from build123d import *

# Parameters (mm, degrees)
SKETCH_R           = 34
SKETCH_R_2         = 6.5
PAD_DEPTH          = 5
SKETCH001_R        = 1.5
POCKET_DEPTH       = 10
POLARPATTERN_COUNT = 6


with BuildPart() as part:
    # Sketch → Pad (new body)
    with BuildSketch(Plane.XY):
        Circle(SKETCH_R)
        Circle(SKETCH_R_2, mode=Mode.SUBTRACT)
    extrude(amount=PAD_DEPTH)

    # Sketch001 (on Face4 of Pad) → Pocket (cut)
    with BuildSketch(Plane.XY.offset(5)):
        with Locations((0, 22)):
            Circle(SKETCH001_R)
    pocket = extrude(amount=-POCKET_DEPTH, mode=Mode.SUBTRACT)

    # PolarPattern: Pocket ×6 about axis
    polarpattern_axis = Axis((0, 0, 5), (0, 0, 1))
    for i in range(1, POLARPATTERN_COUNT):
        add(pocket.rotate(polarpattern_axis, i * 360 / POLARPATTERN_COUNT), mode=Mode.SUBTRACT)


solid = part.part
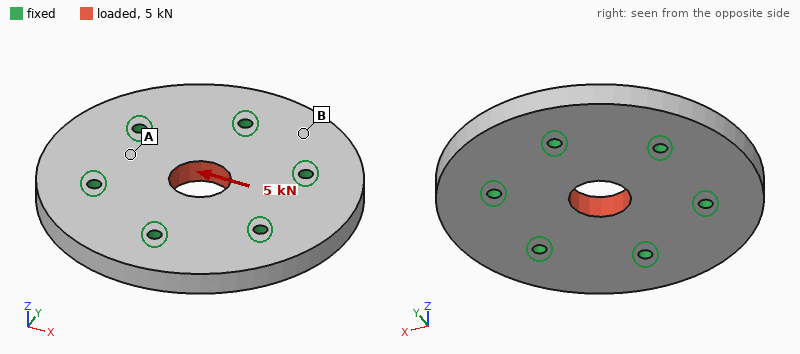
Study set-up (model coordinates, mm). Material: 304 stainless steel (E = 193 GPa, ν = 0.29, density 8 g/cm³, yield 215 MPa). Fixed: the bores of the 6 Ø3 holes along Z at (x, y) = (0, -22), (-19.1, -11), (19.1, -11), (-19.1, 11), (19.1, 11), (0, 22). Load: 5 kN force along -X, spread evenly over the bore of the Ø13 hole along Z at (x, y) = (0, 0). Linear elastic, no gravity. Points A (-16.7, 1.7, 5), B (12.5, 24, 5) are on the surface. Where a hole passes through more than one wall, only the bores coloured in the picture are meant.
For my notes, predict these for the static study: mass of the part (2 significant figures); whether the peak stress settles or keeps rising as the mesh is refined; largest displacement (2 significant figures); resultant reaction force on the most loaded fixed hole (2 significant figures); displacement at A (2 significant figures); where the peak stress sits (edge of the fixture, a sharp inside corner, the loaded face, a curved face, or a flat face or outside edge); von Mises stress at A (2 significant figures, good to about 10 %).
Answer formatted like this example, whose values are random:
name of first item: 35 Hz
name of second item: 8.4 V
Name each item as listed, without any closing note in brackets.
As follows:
mass of the part: 140 g
whether the peak stress settles or keeps rising as the mesh is refined: keeps rising
largest displacement: 1.9 µm
resultant reaction force on the most loaded fixed hole: 1.1 kN
displacement at A: 0.92 µm
where the peak stress sits: edge of the fixture
von Mises stress at A: 11 MPa
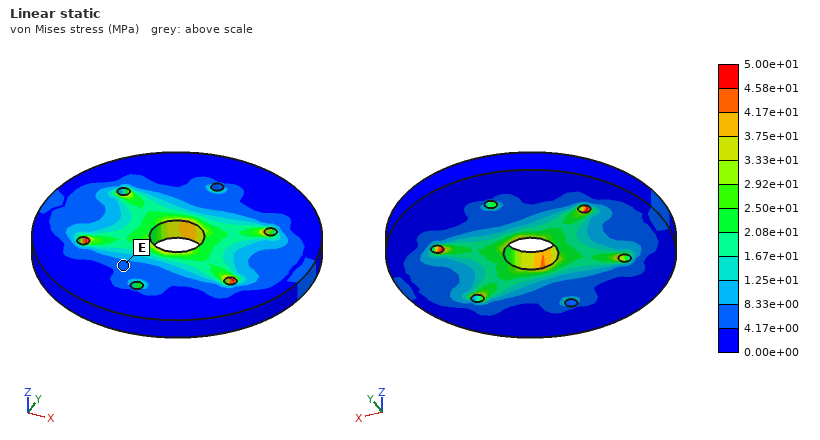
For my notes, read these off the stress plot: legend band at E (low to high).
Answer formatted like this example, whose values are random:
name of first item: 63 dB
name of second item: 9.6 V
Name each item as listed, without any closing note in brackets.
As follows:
legend band at E: 4.17e+00 to 8.33e+00 MPa
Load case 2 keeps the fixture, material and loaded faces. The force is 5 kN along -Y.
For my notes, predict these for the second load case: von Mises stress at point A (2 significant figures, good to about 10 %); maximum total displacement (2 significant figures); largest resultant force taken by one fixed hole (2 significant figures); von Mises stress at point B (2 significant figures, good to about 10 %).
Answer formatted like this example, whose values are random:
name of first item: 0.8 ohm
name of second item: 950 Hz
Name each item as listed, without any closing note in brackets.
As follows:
von Mises stress at point A: 6.7 MPa
maximum total displacement: 1.9 µm
largest resultant force taken by one fixed hole: 1.2 kN
von Mises stress at point B: 4.1 MPa
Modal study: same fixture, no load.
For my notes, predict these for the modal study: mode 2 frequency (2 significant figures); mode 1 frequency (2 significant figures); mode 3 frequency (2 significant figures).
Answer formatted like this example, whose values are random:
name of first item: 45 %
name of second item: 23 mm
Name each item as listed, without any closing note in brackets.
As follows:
mode 2 frequency: 17 kHz
mode 1 frequency: 16 kHz
mode 3 frequency: 17 kHz
